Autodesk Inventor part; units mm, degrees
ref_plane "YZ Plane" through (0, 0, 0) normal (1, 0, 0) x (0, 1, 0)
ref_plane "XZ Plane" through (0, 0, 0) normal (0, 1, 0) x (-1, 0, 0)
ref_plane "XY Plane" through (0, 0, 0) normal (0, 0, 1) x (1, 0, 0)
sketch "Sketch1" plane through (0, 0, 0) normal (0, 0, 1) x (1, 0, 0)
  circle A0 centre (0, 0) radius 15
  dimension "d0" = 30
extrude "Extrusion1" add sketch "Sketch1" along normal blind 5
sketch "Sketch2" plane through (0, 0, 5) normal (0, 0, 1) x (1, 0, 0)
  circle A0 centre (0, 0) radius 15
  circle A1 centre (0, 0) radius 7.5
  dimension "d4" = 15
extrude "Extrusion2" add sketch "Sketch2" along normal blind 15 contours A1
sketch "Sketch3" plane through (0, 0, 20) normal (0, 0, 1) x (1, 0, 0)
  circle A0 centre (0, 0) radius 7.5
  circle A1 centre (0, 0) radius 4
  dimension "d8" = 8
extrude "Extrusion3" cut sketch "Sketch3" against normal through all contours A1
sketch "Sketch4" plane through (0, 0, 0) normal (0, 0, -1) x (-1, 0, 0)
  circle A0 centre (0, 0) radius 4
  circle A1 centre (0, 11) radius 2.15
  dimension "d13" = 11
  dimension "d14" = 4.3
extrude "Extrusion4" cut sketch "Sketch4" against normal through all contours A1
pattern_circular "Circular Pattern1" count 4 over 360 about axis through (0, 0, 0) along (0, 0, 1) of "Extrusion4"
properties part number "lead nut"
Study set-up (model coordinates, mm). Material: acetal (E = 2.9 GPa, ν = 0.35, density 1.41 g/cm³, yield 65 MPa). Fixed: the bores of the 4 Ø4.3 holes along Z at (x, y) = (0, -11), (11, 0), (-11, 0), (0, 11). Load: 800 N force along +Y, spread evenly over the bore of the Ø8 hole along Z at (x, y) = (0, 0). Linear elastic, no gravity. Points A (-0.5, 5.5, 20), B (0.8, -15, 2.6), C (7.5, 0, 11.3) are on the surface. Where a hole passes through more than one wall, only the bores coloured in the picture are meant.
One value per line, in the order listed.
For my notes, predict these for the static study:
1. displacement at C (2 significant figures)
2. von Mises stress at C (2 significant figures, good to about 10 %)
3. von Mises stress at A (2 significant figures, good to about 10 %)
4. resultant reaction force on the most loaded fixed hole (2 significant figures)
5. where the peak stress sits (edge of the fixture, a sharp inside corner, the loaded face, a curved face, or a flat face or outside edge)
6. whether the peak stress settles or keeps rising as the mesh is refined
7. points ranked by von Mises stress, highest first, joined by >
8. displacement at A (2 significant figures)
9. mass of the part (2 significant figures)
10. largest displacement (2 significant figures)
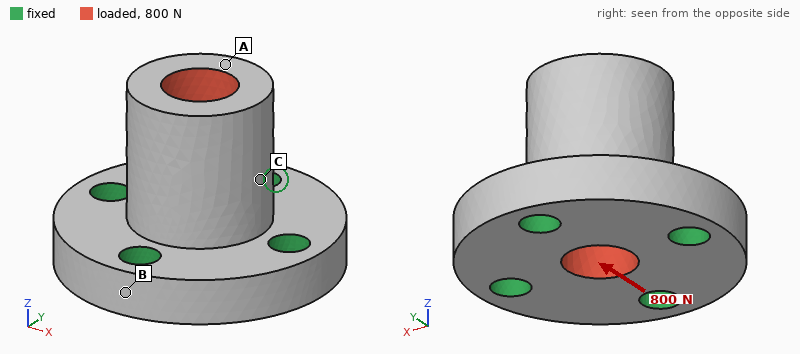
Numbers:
0.072 mm
6.8 MPa
3.8 MPa
400 N
a sharp inside corner
keeps rising
C > A > B
0.16 mm
6.9 g
0.16 mm
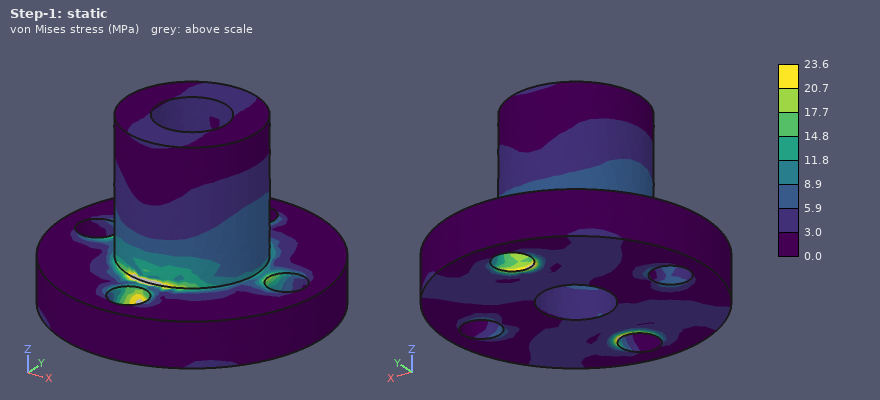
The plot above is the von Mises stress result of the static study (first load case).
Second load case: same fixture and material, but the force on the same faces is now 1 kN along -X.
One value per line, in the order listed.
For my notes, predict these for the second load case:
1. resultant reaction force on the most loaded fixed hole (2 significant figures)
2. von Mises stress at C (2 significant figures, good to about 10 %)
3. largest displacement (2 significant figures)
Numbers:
500 N
5.2 MPa
0.20 mm
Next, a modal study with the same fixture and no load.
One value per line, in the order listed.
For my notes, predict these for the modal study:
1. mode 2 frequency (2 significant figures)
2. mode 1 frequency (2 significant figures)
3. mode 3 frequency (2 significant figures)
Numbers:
6900 Hz
6900 Hz
13 kHz
